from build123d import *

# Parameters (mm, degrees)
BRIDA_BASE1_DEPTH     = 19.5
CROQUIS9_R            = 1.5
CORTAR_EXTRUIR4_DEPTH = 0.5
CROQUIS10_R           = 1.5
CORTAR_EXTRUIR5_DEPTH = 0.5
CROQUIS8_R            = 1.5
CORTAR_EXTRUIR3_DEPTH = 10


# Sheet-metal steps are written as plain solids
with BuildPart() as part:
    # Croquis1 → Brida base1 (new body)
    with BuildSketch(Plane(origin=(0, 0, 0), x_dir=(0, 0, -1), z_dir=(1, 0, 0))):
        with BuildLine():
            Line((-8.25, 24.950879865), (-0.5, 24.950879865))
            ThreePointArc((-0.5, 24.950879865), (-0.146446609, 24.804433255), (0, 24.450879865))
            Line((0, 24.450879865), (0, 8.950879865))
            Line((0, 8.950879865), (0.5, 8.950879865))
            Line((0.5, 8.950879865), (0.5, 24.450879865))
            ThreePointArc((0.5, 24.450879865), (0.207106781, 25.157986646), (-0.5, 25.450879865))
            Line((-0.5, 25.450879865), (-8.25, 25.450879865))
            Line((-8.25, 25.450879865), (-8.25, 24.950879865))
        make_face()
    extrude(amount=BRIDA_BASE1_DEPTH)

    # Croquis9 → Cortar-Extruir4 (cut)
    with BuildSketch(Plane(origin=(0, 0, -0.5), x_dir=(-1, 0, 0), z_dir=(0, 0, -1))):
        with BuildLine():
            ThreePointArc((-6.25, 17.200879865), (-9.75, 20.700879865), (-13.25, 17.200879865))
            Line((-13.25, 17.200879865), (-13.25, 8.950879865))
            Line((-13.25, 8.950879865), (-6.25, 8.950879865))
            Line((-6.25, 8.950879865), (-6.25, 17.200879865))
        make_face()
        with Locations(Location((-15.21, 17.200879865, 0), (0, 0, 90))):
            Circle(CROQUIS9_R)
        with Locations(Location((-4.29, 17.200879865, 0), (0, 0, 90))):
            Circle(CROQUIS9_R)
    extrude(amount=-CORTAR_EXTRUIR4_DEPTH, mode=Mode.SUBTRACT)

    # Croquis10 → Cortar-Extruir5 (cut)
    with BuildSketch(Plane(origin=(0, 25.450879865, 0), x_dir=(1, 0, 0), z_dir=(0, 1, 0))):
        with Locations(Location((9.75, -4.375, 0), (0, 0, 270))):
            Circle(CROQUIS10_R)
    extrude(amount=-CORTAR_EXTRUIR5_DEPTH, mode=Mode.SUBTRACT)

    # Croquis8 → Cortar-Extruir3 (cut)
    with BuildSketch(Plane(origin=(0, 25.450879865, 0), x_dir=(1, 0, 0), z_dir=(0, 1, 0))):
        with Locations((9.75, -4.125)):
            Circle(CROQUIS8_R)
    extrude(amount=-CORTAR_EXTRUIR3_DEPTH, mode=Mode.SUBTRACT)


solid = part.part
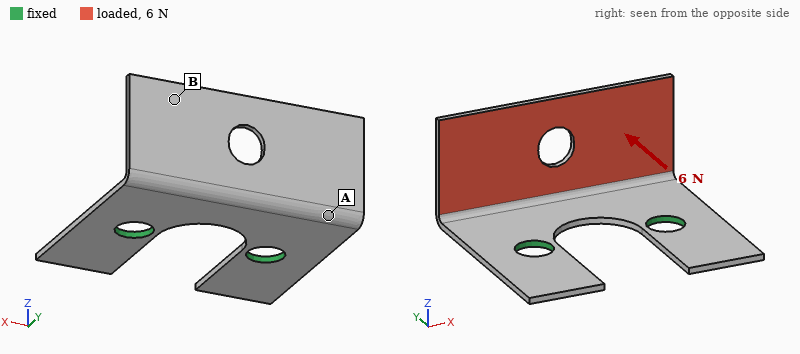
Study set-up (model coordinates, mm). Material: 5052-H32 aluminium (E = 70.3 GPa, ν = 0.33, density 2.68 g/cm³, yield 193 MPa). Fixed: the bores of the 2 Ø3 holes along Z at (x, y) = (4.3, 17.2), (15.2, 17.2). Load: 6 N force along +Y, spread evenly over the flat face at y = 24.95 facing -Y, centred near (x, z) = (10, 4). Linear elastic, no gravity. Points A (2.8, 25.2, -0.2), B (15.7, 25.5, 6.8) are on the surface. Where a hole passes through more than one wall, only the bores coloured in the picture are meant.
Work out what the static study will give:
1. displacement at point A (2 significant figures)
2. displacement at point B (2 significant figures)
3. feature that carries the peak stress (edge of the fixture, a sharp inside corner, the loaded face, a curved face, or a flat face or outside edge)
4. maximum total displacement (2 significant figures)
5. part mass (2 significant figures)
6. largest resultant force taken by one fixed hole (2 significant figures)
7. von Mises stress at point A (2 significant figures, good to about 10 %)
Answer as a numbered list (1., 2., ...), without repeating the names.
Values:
1. 0.054 mm
2. 0.14 mm
3. a flat face or outside edge
4. 0.16 mm
5. 0.51 g
6. 3.1 N
7. 25 MPa
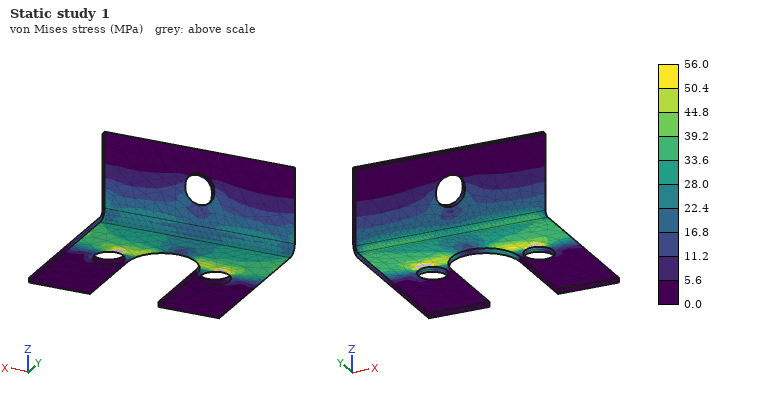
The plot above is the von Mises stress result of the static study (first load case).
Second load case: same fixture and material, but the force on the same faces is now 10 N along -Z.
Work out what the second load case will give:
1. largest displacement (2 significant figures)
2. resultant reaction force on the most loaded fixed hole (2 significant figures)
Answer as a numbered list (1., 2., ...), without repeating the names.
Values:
1. 0.18 mm
2. 5.0 N
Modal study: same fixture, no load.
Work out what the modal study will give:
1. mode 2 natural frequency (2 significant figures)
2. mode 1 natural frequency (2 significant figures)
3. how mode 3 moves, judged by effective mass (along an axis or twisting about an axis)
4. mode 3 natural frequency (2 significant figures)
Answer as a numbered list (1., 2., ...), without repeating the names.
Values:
1. 3900 Hz
2. 2200 Hz
3. along Z
4. 6400 Hz
